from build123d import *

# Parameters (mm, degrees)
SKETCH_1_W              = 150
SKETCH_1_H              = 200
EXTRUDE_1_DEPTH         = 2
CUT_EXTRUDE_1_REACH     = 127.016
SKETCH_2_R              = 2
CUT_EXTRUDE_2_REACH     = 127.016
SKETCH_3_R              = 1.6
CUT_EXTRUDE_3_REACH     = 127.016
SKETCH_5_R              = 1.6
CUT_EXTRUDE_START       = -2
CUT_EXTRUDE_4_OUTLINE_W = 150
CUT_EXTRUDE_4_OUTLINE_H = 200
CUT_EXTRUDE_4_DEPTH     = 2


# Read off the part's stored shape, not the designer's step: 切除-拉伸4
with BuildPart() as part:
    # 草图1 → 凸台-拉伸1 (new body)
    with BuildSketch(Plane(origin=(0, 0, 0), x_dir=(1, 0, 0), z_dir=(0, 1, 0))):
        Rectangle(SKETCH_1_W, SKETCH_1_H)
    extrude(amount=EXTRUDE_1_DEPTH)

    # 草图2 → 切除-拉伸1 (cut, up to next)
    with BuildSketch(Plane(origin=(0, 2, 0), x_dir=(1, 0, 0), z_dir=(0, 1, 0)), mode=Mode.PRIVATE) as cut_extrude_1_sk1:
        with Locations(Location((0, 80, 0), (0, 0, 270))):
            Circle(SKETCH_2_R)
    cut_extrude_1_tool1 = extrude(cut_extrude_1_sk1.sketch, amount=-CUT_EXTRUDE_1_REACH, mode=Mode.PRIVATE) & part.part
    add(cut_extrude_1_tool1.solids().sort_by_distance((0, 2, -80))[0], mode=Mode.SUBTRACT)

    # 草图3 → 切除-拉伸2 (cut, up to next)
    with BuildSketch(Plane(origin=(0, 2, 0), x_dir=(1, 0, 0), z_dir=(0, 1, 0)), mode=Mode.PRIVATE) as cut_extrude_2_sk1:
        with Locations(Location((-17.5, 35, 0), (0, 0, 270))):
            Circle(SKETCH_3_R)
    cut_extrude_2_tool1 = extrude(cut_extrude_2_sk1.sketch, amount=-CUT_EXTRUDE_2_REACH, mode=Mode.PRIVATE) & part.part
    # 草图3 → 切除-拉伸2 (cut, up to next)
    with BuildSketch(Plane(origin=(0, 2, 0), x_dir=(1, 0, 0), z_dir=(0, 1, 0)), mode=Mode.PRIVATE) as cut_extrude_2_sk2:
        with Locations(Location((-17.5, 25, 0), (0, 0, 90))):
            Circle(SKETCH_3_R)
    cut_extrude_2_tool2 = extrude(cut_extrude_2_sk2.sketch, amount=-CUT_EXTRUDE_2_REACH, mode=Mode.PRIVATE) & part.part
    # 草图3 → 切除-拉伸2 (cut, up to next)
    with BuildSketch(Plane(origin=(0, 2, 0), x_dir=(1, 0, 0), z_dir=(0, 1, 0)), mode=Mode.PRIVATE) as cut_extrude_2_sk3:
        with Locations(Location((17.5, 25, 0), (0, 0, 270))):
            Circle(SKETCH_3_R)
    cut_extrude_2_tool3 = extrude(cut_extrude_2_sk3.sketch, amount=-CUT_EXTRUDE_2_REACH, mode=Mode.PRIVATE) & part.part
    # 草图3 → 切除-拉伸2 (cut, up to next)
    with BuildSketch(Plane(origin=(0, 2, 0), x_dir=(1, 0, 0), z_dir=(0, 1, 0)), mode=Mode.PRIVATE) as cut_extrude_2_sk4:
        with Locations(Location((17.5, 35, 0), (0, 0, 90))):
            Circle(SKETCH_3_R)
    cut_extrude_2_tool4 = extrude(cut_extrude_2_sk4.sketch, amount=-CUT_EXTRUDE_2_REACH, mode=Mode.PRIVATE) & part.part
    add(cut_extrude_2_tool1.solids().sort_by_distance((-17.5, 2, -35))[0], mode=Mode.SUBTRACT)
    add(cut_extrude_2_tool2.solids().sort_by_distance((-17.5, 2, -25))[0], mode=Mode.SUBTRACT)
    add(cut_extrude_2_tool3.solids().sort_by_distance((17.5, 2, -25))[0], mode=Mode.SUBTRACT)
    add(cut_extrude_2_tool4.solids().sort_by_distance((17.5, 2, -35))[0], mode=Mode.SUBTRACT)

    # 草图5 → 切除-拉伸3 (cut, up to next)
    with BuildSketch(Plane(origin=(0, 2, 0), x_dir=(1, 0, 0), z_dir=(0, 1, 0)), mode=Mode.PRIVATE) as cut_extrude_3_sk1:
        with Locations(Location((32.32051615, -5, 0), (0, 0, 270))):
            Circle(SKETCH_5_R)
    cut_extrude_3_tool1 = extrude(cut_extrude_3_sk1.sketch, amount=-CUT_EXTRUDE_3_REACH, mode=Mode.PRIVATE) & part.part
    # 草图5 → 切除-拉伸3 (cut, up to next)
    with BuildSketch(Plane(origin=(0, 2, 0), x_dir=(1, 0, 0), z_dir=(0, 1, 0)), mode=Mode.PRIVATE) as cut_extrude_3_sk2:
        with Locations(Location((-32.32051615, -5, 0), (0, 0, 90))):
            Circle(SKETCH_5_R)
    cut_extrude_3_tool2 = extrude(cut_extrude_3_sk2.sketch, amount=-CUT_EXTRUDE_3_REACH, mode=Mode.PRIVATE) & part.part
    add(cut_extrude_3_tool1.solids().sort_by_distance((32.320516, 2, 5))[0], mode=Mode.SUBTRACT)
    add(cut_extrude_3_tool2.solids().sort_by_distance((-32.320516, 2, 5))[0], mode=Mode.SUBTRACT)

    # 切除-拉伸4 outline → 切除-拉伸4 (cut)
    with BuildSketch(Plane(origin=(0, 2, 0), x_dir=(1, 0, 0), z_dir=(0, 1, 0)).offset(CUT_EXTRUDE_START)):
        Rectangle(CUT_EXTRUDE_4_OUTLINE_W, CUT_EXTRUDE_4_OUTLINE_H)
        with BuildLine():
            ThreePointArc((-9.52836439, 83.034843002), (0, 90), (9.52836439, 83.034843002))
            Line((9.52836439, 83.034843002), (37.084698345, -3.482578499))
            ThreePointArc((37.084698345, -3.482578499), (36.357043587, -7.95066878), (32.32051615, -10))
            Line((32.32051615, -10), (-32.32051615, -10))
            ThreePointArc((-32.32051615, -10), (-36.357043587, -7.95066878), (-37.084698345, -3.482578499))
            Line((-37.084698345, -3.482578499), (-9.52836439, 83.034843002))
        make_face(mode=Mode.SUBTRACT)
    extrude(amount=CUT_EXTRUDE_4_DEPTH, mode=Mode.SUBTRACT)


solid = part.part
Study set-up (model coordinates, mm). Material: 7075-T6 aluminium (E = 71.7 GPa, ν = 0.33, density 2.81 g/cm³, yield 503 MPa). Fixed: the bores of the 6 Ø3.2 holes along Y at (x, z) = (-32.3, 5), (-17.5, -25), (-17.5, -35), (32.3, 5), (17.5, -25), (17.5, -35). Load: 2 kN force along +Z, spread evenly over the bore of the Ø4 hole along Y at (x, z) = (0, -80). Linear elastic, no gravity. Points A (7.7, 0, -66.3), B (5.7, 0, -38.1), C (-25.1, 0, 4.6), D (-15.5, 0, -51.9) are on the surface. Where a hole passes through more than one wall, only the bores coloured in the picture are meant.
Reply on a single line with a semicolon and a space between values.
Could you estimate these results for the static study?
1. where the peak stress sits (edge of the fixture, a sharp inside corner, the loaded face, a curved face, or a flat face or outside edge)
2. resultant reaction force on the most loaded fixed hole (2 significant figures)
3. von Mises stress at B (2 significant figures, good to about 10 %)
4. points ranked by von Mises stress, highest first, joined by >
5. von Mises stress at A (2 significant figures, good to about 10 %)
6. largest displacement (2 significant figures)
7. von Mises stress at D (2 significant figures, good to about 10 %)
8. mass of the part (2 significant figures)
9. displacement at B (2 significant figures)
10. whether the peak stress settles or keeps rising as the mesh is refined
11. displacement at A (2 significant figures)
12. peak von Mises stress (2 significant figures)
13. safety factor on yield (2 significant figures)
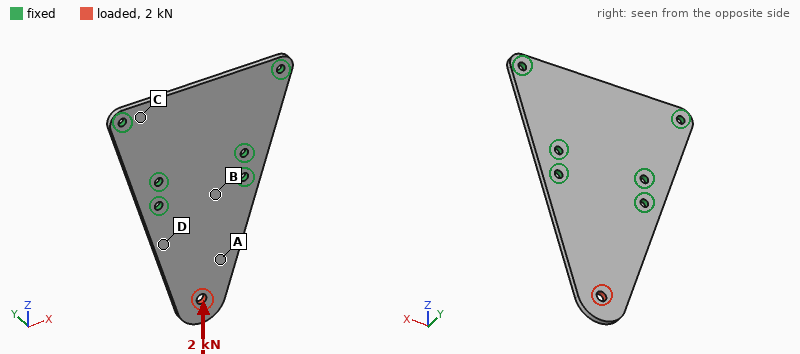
the loaded face; 680 N; 16 MPa; A > D > B > C; 36 MPa; 29 µm; 28 MPa; 26 g; 4.6 µm; settles; 14 µm; 160 MPa; 3.2
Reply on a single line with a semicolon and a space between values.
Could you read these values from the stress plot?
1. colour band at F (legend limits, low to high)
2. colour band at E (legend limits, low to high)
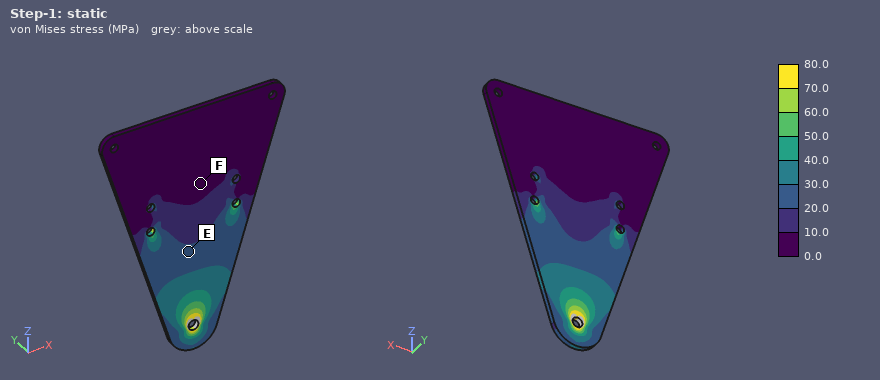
0.0 to 10.0 MPa; 20.0 to 30.0 MPa
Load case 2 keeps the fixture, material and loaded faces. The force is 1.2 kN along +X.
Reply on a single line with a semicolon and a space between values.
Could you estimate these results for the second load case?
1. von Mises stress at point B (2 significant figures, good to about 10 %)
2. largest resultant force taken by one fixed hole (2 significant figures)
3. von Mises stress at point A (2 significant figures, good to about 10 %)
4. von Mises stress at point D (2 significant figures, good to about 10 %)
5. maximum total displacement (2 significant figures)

14 MPa; 1.3 kN; 42 MPa; 59 MPa; 98 µm
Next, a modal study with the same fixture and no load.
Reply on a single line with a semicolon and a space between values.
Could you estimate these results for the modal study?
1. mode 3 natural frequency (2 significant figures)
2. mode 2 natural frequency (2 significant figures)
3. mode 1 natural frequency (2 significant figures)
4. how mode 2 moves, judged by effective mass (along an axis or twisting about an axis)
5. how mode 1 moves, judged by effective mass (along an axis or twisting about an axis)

3300 Hz; 3100 Hz; 760 Hz; along Y; along Y
